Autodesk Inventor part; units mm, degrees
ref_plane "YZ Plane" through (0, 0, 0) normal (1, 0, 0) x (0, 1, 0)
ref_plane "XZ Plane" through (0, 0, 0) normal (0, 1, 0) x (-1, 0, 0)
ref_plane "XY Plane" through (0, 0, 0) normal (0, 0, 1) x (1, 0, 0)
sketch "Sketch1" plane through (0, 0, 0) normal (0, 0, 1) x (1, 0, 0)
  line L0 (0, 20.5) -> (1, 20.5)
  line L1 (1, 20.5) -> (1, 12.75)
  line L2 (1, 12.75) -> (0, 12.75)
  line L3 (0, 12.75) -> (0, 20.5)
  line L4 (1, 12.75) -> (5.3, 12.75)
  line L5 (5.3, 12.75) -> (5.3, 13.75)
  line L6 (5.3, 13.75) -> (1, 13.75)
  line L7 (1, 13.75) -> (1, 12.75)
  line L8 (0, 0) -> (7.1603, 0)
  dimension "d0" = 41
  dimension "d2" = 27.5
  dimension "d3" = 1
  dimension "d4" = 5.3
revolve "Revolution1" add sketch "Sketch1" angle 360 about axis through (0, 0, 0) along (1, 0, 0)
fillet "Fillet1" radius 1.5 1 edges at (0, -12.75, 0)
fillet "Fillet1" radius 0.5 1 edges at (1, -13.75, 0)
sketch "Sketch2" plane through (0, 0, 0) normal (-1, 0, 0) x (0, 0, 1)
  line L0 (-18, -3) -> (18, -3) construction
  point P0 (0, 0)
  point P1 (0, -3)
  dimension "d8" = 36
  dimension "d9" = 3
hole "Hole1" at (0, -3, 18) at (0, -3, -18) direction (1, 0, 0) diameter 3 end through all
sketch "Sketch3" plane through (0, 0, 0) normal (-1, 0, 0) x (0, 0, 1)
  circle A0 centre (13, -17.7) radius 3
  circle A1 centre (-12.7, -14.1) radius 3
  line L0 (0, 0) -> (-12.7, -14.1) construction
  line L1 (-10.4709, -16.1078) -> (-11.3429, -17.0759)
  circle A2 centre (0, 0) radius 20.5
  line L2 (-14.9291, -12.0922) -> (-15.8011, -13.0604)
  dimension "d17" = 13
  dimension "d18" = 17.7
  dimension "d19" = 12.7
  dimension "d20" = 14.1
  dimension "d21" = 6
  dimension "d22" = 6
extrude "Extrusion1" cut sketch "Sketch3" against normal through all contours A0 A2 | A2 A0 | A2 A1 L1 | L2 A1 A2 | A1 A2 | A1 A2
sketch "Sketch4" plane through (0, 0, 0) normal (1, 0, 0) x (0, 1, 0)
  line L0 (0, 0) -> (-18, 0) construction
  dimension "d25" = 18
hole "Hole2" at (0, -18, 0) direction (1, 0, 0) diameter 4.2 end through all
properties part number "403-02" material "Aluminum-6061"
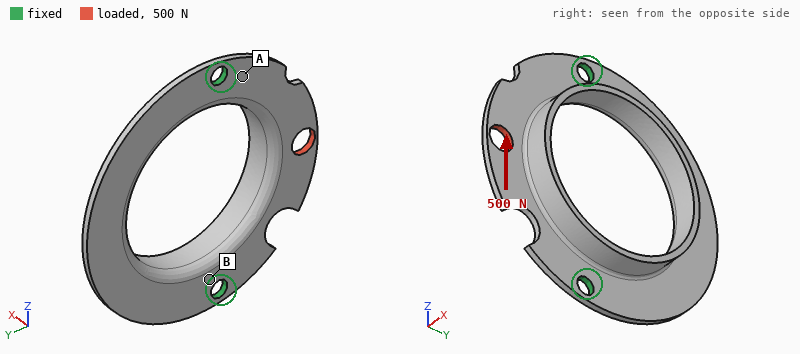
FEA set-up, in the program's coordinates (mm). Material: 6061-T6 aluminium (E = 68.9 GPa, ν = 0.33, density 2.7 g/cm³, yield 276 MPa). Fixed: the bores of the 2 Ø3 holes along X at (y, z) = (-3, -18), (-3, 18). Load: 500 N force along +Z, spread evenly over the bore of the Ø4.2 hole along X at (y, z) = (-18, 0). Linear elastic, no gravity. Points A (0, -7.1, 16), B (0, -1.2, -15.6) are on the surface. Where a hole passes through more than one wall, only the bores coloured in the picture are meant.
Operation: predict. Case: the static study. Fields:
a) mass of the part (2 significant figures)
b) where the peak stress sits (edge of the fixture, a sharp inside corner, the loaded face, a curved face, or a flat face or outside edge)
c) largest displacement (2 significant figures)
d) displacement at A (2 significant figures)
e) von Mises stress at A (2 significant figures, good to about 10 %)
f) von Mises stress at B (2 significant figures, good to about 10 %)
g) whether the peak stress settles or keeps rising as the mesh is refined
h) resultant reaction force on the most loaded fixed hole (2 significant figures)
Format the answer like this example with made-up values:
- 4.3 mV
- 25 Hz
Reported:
- 2.9 g
- a sharp inside corner
- 35 µm
- 7.2 µm
- 58 MPa
- 15 MPa
- keeps rising
- 320 N
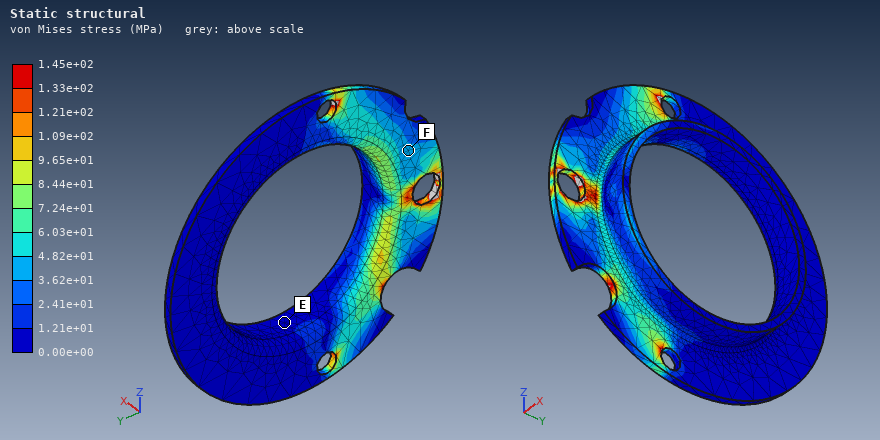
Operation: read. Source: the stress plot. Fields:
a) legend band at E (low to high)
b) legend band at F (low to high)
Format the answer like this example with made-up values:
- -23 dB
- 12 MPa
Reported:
- 0.00e+00 to 1.21e+01 MPa
- 3.62e+01 to 4.82e+01 MPa
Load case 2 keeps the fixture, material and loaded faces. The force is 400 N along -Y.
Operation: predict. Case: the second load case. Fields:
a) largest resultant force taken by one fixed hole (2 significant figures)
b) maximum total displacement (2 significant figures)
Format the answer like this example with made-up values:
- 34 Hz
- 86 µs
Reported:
- 270 N
- 58 µm
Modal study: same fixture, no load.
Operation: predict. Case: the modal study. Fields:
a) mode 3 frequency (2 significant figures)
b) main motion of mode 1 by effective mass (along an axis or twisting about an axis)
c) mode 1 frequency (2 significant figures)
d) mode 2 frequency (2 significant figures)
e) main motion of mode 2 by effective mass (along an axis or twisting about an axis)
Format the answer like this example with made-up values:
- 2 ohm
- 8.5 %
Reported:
- 5300 Hz
- along X
- 1800 Hz
- 3600 Hz
- along X
